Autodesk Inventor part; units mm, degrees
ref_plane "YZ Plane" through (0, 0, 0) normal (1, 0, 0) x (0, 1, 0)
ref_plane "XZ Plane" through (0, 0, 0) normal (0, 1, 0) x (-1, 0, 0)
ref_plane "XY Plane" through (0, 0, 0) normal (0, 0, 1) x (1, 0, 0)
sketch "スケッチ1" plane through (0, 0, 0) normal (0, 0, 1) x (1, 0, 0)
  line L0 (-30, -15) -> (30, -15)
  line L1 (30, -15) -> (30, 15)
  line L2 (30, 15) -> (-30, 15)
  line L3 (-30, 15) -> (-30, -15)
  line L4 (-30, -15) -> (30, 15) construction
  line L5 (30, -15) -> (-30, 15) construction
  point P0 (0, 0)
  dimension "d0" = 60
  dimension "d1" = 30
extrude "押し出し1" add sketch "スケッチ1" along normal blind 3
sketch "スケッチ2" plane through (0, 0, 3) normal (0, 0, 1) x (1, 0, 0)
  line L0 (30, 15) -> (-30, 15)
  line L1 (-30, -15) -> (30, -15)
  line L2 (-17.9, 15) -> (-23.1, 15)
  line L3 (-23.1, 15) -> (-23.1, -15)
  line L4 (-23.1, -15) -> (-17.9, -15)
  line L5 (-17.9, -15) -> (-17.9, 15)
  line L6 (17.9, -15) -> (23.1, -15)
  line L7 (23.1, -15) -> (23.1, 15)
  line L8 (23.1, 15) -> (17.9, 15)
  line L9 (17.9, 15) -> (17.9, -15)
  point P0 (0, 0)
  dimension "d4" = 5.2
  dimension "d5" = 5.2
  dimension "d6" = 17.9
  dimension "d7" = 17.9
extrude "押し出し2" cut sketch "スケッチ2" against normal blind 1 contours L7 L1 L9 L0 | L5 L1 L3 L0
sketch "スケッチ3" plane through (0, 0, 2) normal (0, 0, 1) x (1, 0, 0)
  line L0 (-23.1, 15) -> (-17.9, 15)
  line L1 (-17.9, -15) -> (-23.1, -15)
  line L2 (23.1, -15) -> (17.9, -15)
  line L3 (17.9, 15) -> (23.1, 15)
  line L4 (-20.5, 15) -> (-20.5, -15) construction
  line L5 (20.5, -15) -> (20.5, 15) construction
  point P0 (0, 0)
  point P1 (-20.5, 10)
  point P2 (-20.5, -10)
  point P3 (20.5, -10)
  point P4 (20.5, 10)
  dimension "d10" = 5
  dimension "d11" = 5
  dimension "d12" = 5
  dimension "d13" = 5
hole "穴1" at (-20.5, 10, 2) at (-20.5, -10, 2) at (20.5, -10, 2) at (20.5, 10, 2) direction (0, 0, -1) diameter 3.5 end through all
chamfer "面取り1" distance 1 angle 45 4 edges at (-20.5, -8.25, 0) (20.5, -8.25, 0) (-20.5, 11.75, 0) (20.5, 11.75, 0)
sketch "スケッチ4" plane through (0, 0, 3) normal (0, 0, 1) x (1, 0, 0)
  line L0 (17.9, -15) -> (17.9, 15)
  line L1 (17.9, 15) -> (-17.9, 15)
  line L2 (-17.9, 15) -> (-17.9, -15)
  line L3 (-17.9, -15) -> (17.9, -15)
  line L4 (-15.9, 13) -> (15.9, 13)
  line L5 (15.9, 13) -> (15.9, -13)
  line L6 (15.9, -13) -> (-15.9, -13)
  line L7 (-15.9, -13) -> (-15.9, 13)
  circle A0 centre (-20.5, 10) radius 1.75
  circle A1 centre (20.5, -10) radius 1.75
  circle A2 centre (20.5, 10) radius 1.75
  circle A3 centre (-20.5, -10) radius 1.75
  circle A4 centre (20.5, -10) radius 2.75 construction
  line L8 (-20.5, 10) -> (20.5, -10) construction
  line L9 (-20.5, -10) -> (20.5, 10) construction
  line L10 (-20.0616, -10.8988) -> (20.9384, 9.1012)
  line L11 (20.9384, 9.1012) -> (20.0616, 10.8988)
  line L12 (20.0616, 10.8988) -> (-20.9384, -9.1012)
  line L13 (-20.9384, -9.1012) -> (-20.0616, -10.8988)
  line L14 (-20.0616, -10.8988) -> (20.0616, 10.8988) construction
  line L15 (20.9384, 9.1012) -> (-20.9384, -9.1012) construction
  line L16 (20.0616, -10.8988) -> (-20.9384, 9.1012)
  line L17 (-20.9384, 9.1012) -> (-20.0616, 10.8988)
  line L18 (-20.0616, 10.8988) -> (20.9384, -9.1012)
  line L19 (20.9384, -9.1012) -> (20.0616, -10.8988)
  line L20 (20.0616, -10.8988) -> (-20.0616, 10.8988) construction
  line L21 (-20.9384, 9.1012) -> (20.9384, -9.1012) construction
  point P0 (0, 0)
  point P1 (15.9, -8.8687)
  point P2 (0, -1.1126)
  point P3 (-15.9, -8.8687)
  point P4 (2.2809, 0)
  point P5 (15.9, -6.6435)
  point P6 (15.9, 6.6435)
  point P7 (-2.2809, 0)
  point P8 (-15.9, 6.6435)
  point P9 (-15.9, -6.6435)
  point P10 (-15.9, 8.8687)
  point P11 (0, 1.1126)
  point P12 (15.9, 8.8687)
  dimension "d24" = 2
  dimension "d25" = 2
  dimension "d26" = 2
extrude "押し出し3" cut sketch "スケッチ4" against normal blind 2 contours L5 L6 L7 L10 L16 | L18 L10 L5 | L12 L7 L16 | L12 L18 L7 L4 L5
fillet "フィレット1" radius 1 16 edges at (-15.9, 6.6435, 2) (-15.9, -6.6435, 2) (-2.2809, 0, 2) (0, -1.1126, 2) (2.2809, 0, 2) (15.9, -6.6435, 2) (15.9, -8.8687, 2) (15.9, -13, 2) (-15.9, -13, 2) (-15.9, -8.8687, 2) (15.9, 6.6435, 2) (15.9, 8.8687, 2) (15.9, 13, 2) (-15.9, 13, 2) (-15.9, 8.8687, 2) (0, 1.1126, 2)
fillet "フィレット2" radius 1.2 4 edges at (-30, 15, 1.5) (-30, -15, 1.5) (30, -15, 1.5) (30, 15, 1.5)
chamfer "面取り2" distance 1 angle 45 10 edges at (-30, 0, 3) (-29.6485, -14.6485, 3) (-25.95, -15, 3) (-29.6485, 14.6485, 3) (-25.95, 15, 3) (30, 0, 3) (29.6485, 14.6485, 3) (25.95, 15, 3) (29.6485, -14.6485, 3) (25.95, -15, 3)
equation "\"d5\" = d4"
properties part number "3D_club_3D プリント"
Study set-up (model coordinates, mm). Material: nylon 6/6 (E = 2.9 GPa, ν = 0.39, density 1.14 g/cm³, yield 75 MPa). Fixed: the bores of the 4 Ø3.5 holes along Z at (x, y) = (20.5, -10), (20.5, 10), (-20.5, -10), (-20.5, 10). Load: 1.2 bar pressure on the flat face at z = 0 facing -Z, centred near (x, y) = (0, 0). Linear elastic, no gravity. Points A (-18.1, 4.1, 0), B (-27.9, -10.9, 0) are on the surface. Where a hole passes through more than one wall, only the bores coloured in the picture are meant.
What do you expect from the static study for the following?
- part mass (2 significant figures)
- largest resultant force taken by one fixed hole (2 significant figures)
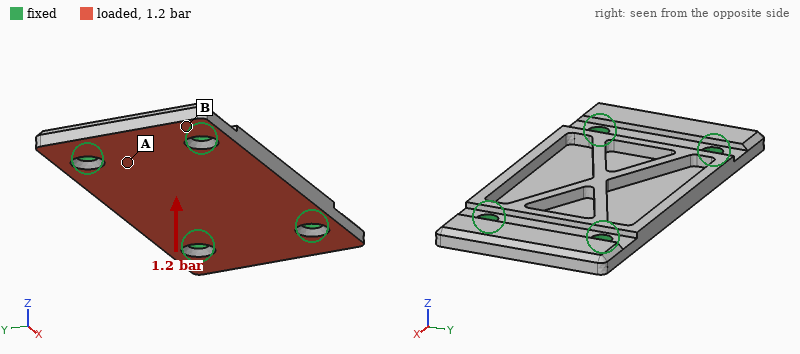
4.1 g
58 N
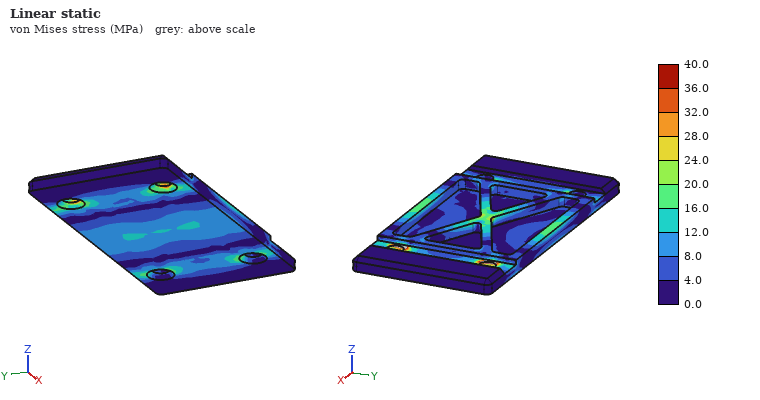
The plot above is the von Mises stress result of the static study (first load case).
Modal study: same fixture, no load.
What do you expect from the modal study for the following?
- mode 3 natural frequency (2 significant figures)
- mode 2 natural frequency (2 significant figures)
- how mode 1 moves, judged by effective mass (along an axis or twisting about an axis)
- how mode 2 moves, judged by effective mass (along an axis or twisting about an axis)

3700 Hz
2800 Hz
along Z
twisting about X
